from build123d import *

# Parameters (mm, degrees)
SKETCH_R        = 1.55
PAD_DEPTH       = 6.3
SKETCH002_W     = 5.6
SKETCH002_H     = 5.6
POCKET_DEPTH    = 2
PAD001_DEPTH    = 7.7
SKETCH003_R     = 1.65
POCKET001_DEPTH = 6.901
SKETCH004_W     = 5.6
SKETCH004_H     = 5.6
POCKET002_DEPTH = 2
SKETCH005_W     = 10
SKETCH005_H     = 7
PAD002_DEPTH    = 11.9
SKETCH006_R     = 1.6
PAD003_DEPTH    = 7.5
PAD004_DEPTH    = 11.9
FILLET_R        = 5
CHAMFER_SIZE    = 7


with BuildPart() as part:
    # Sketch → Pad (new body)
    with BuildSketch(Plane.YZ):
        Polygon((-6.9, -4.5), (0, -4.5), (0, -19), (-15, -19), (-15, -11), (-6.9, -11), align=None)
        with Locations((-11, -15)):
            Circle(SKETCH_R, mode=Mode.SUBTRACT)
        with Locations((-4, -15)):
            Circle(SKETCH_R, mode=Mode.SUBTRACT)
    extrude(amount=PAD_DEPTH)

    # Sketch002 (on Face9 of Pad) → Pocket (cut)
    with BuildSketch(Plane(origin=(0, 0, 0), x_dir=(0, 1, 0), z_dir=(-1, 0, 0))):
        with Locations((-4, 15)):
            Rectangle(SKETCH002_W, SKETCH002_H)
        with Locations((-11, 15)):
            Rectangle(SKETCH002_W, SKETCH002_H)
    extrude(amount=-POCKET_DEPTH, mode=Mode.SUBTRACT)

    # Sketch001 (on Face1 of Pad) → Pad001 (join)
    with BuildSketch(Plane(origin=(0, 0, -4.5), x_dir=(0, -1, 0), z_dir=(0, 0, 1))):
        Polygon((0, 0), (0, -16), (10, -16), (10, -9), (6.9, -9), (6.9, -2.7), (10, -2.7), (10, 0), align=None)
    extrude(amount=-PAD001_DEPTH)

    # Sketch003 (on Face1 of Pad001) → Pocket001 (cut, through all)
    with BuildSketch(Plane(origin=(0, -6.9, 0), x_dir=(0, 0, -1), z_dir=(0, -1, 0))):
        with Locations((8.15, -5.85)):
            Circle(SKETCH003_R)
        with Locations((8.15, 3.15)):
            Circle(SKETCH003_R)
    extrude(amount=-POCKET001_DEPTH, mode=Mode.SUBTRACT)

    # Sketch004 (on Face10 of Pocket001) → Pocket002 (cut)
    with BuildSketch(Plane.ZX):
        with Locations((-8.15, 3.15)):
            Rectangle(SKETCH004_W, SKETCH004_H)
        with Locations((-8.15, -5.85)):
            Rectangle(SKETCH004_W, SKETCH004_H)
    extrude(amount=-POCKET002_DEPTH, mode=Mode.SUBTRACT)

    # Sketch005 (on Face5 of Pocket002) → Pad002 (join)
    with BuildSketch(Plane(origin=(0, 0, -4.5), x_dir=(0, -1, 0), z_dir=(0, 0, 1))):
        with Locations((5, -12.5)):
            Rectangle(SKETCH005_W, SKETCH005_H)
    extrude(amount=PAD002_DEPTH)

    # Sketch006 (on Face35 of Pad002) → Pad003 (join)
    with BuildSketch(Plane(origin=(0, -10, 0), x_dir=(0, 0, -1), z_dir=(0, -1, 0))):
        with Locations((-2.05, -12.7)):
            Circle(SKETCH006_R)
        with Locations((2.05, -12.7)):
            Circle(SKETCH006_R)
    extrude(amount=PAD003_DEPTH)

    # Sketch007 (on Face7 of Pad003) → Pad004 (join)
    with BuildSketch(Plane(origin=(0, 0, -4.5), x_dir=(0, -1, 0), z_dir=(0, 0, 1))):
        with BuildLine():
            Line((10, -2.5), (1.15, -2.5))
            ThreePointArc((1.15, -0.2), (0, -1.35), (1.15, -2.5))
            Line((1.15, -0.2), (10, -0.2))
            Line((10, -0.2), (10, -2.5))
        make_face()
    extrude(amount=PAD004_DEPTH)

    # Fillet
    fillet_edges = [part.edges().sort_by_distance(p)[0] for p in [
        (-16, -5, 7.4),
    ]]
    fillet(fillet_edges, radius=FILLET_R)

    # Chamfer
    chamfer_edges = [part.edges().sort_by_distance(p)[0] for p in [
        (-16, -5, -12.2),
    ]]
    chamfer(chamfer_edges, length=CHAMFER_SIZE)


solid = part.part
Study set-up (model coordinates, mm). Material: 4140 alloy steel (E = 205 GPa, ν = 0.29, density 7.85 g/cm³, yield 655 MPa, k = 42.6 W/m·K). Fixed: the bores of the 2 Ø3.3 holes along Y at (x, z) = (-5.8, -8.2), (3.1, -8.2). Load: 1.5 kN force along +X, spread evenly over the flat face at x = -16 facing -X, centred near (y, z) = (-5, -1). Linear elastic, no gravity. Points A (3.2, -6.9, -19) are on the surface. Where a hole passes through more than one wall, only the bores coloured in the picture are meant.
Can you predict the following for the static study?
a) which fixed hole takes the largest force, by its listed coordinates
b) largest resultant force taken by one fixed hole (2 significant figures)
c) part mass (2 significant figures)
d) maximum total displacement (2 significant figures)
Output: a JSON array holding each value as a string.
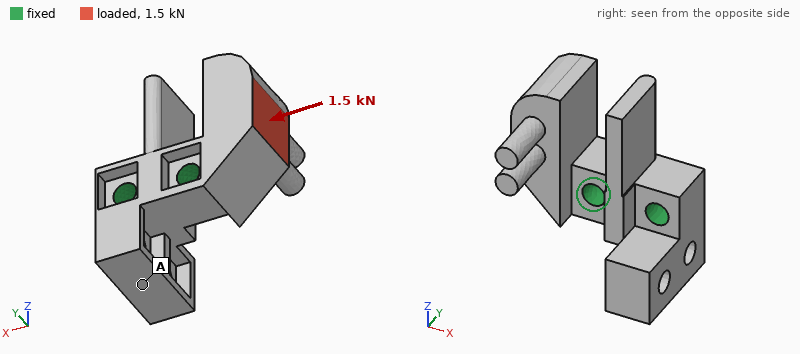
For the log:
["(-5.8, -8.2)", "1.5 kN", "21 g", "40 µm"]
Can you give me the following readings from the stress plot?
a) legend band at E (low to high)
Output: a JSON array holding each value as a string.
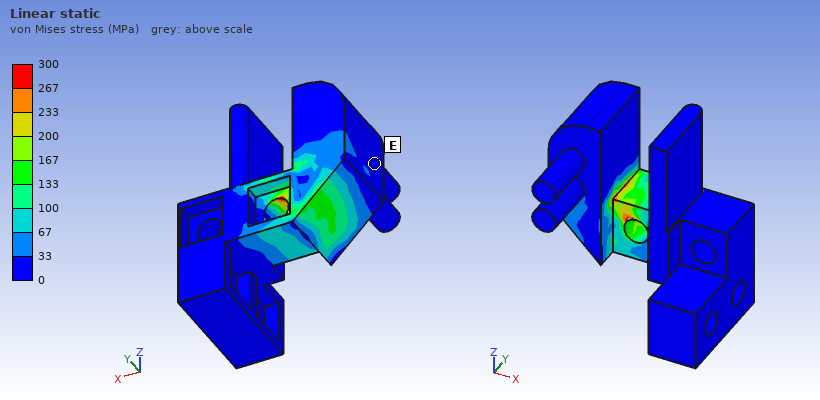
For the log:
["0 to 33 MPa"]
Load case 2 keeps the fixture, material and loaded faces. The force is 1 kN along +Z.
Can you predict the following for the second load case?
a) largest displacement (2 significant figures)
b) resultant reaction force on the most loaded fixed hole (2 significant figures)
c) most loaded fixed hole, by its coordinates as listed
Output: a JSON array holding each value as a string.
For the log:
["31 µm", "1.4 kN", "(-5.8, -8.2)"]
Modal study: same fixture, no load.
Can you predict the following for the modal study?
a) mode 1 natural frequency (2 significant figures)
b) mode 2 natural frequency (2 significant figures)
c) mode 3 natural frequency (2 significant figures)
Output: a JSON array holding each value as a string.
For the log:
["11 kHz", "11 kHz", "11 kHz"]
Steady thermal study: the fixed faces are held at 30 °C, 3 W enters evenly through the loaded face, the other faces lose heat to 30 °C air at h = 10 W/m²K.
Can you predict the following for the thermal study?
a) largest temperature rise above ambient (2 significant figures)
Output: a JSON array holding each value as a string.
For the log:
["15 K"]
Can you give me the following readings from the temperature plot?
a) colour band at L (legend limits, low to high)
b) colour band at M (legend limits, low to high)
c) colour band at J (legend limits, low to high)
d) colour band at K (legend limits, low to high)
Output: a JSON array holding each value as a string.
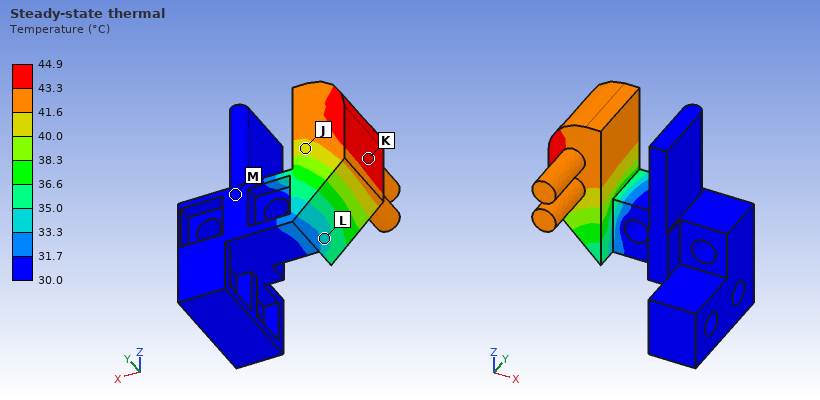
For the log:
["33.3 to 35.0 °C", "30.0 to 31.7 °C", "40.0 to 41.6 °C", "43.3 to 44.9 °C"]
